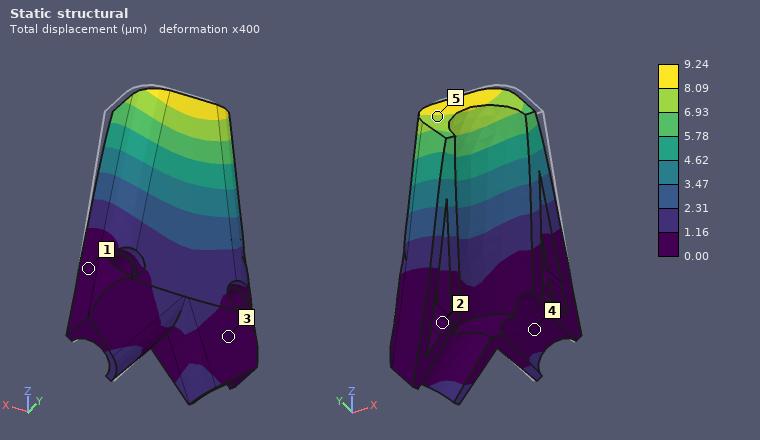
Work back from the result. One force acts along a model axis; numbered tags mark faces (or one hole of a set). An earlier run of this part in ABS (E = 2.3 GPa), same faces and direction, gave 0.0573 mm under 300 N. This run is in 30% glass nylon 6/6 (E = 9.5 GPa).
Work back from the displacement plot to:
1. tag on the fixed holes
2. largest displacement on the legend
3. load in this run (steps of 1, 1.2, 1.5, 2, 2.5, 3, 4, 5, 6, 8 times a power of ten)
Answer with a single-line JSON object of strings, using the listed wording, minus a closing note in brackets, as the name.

{"tag on the fixed holes": "2", "largest displacement on the legend": "9.24 µm", "load in this run": "200 N"}
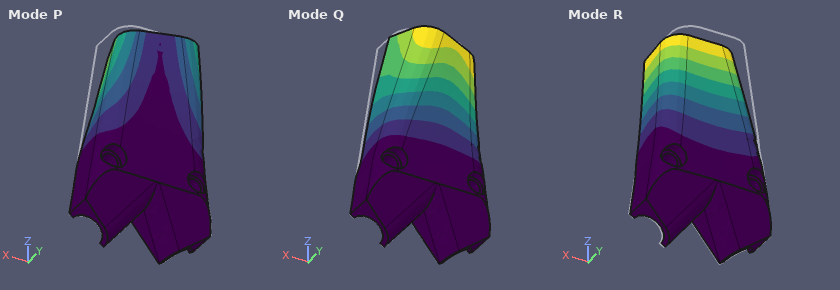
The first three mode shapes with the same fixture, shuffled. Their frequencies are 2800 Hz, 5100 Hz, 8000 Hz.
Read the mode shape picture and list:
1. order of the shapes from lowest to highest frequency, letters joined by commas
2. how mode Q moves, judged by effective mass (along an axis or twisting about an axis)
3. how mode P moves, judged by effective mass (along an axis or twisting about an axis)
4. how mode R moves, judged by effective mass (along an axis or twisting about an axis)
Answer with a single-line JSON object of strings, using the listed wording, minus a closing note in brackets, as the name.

{"order of the shapes from lowest to highest frequency, letters joined by commas": "R, P, Q", "how mode Q moves, judged by effective mass": "along X", "how mode P moves, judged by effective mass": "along X", "how mode R moves, judged by effective mass": "along Y"}
